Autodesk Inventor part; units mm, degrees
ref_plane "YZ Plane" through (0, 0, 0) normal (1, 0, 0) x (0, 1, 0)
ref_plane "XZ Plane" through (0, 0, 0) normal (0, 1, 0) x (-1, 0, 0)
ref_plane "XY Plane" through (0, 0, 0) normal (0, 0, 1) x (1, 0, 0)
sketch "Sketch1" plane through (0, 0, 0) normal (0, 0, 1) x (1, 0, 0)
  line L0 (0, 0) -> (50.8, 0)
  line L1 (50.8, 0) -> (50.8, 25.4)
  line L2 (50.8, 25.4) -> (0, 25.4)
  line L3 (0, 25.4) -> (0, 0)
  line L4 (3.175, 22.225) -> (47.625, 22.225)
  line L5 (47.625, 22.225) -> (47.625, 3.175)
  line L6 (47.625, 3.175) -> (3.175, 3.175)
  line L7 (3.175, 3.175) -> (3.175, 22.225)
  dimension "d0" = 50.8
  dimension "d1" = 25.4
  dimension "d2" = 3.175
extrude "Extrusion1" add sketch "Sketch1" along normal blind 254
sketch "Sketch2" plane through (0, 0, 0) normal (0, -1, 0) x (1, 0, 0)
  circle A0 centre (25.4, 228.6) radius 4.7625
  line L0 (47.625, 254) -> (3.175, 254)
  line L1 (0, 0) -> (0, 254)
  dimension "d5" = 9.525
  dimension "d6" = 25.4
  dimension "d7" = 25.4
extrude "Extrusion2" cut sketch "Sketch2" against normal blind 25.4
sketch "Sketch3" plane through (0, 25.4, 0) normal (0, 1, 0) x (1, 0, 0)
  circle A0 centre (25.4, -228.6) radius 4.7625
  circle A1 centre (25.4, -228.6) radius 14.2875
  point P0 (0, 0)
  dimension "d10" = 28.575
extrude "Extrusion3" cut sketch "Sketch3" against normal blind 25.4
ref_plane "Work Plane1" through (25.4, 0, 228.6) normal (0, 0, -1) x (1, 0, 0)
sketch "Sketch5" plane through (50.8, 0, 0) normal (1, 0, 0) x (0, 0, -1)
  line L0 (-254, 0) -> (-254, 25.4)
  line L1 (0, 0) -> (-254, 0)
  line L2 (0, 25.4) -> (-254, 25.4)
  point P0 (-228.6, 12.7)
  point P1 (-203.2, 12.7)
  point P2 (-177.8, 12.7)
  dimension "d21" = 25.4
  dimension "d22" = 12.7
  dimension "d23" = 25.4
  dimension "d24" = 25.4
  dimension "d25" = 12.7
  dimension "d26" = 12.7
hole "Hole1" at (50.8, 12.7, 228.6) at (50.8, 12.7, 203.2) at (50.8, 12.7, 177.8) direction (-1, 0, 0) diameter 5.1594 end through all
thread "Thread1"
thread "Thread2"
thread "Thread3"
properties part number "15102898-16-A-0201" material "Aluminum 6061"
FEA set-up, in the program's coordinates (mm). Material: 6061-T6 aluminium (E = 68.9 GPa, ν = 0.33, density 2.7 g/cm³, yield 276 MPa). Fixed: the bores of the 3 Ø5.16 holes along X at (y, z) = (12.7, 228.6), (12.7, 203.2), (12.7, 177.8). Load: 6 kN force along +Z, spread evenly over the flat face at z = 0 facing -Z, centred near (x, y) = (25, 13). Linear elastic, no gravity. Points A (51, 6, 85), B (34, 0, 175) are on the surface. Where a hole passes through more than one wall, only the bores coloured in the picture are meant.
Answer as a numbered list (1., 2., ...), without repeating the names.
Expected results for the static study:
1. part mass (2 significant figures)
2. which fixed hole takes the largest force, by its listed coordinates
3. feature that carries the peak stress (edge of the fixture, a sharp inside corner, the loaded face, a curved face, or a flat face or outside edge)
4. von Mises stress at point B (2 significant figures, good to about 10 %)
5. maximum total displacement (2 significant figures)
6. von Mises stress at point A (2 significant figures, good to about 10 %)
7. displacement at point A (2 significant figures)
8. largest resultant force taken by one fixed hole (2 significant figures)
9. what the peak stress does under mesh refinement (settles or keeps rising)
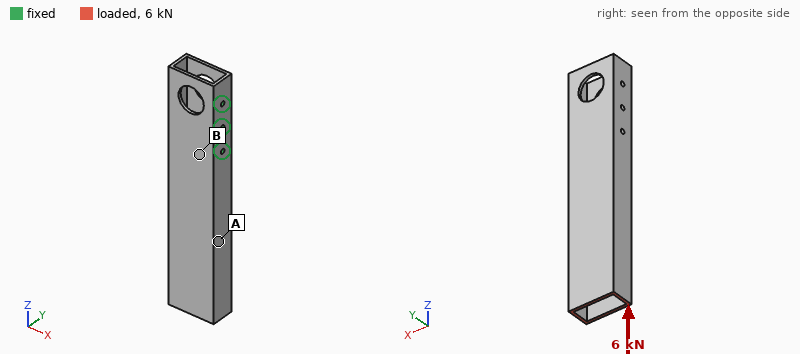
1. 290 g
2. (12.7, 177.8)
3. edge of the fixture
4. 30 MPa
5. 0.62 mm
6. 14 MPa
7. 0.34 mm
8. 3.7 kN
9. keeps rising
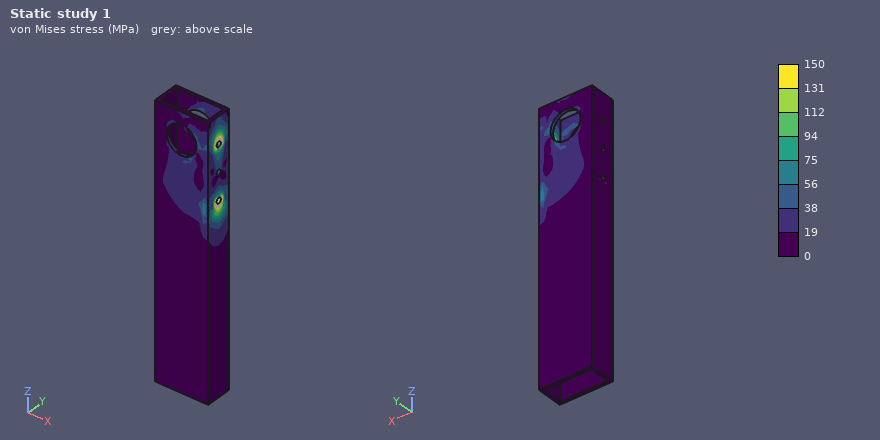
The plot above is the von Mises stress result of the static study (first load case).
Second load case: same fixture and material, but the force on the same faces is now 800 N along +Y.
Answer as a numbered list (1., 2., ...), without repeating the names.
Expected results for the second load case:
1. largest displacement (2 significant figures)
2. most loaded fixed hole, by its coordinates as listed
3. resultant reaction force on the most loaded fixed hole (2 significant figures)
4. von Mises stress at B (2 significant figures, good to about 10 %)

1. 1.4 mm
2. (12.7, 177.8)
3. 3.8 kN
4. 54 MPa
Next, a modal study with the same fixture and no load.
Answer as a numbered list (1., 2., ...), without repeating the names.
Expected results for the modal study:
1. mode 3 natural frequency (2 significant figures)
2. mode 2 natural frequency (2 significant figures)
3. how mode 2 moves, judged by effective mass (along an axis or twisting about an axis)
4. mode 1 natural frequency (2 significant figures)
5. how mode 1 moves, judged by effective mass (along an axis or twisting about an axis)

1. 770 Hz
2. 550 Hz
3. along X
4. 440 Hz
5. along Y
